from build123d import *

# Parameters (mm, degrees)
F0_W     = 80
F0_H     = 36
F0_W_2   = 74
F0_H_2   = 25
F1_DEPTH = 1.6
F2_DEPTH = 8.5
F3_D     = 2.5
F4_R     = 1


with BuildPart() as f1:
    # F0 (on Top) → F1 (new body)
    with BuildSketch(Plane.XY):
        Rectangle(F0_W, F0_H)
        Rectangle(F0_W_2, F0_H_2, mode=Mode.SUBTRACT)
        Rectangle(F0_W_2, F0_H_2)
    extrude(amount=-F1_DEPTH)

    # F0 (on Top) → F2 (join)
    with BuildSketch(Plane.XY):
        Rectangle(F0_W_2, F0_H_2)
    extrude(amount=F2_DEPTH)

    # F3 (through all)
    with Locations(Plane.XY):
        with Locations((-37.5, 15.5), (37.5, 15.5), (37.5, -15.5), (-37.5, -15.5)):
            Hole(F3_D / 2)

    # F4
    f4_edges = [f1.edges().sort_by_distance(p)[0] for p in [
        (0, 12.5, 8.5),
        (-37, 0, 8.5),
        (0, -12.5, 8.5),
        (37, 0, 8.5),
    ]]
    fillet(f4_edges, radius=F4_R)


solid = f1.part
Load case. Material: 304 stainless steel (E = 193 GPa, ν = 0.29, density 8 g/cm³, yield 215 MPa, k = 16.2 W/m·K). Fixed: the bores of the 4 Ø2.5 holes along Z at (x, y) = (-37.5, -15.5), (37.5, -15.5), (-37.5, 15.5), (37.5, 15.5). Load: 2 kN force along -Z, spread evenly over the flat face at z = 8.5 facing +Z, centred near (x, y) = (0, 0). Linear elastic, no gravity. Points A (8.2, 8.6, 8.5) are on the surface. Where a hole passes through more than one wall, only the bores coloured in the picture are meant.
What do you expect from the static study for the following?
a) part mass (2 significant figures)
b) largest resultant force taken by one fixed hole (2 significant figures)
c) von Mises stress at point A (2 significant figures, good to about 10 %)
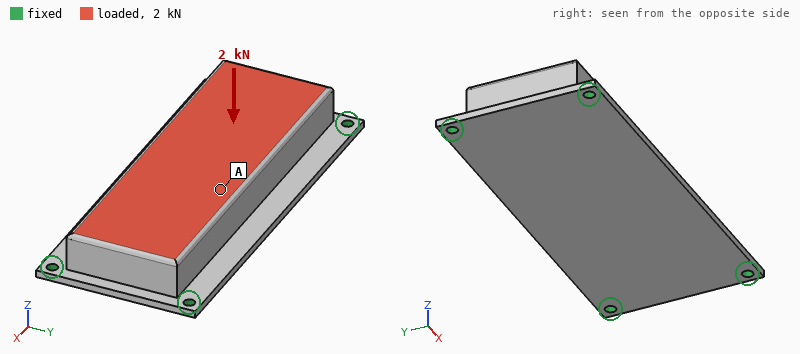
160 g
830 N
32 MPa
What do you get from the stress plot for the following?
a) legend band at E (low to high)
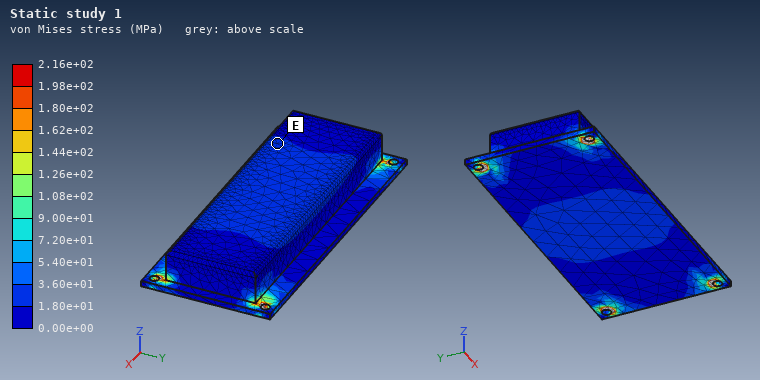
1.80e+01 to 3.60e+01 MPa
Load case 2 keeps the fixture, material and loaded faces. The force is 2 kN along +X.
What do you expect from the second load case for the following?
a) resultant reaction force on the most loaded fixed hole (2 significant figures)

560 N
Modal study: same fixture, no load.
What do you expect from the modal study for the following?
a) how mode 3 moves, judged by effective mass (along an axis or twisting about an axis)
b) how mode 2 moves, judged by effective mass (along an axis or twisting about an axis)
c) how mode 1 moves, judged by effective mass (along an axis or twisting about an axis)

twisting about Y
along Y
along Z
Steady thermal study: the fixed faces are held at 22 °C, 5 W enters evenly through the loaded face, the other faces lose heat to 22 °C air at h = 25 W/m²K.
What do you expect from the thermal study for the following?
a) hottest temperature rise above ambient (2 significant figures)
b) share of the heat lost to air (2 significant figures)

21 K
49 %
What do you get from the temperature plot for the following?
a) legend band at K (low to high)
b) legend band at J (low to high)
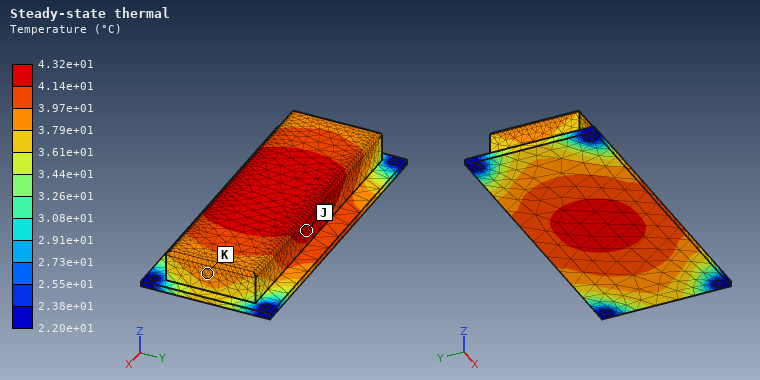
3.79e+01 to 3.97e+01 °C
4.14e+01 to 4.32e+01 °C
